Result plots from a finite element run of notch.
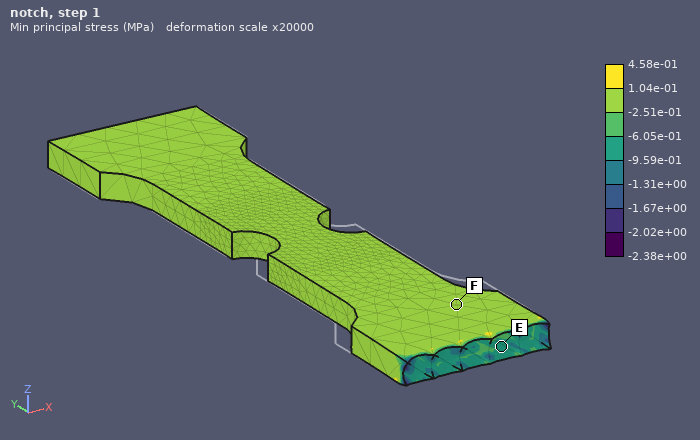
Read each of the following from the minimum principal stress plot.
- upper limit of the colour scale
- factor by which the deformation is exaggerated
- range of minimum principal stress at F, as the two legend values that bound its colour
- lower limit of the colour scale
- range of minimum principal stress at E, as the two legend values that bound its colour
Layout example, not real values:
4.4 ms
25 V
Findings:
4.58e-01 MPa
20000
-2.51e-01 to 1.04e-01 MPa
-2.38e+00 MPa
-9.59e-01 to -6.05e-01 MPa
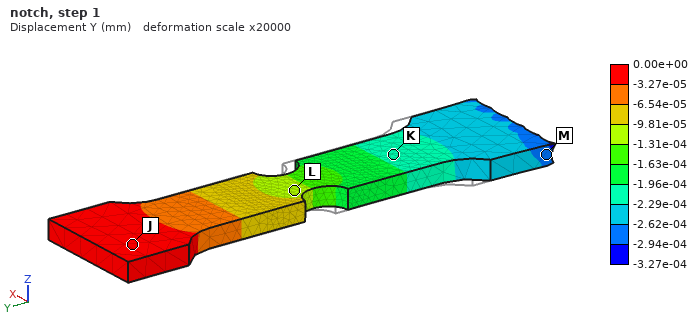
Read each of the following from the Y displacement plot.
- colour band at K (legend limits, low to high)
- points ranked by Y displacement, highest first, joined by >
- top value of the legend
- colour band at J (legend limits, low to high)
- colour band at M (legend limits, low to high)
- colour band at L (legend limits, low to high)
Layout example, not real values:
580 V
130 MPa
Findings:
-2.29e-04 to -1.96e-04 mm
J > L > K > M
0.00e+00 mm
-3.27e-05 to 0.00e+00 mm
-2.94e-04 to -2.62e-04 mm
-1.31e-04 to -9.81e-05 mm
